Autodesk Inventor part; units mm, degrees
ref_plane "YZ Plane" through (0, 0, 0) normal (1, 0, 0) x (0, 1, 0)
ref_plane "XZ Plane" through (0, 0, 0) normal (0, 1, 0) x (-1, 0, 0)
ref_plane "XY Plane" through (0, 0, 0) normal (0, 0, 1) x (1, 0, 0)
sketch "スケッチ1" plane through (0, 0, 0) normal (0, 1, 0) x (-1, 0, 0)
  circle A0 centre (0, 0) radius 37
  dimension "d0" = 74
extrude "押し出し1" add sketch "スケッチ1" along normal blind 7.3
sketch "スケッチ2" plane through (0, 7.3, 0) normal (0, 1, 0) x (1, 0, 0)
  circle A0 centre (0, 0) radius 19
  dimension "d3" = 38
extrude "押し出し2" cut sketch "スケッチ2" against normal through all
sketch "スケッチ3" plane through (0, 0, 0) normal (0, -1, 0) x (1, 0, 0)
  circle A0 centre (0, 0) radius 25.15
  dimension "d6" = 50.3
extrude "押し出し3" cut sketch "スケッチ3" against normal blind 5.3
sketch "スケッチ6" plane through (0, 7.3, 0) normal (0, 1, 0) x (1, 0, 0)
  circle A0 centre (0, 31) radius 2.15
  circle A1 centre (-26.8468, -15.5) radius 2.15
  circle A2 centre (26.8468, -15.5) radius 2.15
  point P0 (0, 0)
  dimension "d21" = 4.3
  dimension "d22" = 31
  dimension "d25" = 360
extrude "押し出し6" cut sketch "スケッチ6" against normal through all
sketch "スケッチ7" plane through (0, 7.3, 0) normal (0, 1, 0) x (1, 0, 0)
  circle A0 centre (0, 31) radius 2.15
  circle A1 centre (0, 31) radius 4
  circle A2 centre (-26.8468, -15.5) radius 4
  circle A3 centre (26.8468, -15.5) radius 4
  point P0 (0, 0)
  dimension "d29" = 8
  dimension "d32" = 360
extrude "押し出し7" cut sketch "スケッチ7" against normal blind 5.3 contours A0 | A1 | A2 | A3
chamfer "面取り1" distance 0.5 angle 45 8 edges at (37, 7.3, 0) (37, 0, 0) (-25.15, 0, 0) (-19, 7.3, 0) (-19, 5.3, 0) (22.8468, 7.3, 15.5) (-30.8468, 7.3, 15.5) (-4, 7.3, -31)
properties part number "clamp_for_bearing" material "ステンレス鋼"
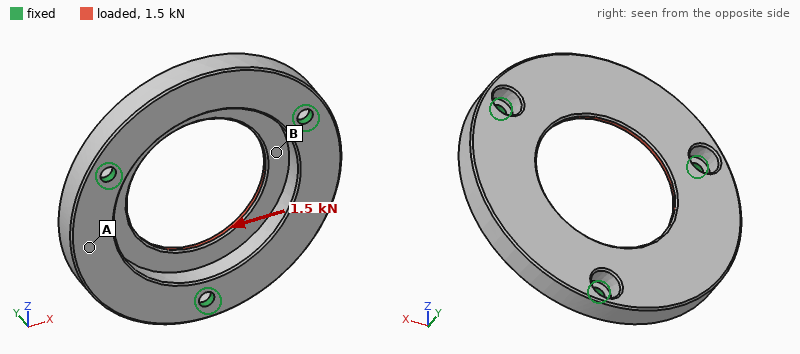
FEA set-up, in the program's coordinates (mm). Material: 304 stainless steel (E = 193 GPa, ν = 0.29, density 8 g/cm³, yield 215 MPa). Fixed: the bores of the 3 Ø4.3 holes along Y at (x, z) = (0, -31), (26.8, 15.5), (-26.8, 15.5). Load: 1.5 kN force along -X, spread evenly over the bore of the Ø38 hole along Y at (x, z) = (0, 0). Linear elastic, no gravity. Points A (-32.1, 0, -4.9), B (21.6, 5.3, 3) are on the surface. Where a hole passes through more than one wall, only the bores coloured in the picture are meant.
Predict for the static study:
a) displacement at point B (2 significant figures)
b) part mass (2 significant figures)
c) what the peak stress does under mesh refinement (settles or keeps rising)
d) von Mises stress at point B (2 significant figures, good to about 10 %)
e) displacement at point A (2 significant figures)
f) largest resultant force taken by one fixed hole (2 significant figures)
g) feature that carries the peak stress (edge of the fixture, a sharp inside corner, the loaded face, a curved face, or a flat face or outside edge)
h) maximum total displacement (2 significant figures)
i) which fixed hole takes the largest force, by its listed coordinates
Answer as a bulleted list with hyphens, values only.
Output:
- 2.3 µm
- 140 g
- keeps rising
- 8.6 MPa
- 4.8 µm
- 570 N
- edge of the fixture
- 8.3 µm
- (0, -31)
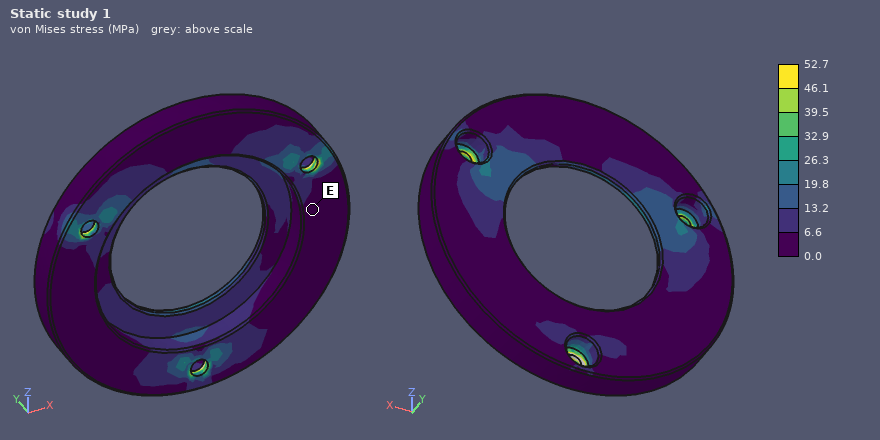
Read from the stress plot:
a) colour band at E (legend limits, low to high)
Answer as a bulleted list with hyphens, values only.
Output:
- 0.0 to 6.6 MPa
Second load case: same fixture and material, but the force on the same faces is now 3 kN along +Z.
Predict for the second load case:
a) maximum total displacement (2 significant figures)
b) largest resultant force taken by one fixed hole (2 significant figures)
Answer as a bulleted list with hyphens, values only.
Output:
- 19 µm
- 1.1 kN
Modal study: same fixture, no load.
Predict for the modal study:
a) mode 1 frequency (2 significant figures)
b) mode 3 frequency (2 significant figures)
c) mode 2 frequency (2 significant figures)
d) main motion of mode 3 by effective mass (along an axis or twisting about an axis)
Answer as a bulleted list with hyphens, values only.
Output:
- 4400 Hz
- 6700 Hz
- 4400 Hz
- along Y
